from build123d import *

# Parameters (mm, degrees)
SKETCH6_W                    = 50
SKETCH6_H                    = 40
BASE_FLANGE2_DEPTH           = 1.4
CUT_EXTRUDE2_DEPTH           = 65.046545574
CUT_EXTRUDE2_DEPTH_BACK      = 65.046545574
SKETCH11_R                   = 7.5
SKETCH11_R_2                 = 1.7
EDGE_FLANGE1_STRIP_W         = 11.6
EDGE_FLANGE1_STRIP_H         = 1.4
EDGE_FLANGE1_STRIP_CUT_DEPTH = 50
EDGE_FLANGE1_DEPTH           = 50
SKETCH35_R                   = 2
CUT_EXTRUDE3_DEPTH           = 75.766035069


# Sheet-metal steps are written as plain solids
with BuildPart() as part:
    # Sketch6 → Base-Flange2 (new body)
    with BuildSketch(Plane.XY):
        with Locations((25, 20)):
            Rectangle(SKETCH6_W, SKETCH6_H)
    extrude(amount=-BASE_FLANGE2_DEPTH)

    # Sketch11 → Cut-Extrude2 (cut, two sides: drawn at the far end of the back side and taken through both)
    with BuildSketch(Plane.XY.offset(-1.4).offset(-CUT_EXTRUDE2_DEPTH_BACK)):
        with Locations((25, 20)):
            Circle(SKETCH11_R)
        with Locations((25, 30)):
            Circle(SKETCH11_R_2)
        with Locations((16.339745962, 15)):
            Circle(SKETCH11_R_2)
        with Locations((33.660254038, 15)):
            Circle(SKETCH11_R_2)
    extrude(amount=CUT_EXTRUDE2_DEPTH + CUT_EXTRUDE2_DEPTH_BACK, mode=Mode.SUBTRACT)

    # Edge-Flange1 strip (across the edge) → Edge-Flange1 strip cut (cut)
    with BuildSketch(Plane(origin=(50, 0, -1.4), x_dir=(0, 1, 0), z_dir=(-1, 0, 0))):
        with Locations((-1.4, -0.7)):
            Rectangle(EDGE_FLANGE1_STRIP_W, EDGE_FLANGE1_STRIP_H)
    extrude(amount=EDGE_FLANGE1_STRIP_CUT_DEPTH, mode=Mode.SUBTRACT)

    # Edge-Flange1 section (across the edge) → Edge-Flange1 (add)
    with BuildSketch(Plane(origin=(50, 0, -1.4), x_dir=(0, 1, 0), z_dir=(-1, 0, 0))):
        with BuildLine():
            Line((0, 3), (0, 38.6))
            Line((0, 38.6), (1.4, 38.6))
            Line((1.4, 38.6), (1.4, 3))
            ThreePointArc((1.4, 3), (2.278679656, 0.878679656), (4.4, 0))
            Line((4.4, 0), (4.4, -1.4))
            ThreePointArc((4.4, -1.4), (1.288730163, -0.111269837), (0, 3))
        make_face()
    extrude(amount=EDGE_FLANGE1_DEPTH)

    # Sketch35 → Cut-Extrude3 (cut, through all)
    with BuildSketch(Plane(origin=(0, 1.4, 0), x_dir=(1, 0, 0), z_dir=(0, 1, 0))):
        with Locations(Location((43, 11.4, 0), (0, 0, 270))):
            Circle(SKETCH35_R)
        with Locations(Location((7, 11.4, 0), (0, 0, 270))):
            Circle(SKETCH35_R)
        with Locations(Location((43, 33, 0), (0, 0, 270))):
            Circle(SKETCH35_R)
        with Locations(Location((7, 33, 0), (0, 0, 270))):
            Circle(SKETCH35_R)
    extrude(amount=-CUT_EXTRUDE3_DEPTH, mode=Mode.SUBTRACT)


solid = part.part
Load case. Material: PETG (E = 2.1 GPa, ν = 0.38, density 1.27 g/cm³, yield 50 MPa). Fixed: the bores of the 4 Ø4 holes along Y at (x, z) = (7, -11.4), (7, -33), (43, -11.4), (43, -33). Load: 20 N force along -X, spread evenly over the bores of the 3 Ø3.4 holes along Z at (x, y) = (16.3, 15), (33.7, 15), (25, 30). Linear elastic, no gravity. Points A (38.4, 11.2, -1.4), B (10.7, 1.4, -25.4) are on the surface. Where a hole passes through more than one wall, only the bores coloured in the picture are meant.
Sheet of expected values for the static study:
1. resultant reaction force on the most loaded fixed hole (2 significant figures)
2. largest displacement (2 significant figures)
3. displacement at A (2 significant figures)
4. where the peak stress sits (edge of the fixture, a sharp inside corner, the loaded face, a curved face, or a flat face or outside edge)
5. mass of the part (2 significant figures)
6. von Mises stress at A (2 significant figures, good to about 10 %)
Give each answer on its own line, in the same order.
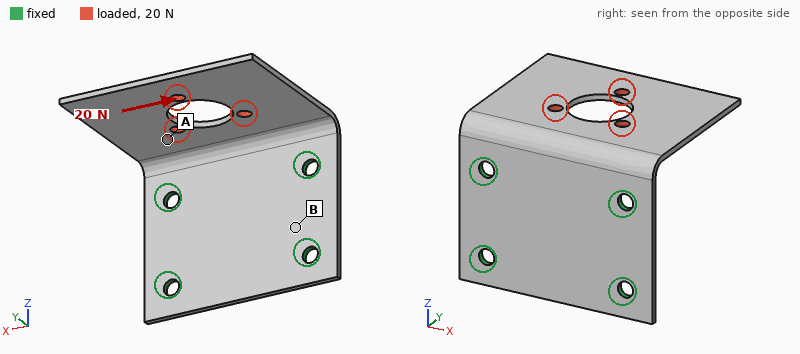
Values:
15 N
0.88 mm
0.28 mm
a flat face or outside edge
6.4 g
2.3 MPa
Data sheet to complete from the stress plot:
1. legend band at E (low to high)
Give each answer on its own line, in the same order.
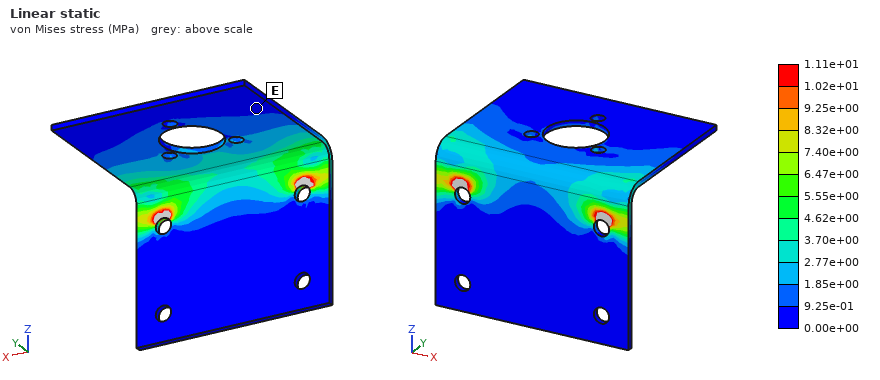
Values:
0.00e+00 to 9.25e-01 MPa
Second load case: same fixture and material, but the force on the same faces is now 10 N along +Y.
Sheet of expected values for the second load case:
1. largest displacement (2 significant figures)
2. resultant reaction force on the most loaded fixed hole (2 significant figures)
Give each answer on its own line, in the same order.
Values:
0.87 mm
5.6 N
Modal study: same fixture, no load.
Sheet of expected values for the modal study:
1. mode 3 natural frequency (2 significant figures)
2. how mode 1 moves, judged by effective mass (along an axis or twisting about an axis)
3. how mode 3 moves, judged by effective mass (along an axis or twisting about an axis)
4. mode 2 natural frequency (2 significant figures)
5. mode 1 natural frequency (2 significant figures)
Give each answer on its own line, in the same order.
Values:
620 Hz
along Z
along X
310 Hz
140 Hz
